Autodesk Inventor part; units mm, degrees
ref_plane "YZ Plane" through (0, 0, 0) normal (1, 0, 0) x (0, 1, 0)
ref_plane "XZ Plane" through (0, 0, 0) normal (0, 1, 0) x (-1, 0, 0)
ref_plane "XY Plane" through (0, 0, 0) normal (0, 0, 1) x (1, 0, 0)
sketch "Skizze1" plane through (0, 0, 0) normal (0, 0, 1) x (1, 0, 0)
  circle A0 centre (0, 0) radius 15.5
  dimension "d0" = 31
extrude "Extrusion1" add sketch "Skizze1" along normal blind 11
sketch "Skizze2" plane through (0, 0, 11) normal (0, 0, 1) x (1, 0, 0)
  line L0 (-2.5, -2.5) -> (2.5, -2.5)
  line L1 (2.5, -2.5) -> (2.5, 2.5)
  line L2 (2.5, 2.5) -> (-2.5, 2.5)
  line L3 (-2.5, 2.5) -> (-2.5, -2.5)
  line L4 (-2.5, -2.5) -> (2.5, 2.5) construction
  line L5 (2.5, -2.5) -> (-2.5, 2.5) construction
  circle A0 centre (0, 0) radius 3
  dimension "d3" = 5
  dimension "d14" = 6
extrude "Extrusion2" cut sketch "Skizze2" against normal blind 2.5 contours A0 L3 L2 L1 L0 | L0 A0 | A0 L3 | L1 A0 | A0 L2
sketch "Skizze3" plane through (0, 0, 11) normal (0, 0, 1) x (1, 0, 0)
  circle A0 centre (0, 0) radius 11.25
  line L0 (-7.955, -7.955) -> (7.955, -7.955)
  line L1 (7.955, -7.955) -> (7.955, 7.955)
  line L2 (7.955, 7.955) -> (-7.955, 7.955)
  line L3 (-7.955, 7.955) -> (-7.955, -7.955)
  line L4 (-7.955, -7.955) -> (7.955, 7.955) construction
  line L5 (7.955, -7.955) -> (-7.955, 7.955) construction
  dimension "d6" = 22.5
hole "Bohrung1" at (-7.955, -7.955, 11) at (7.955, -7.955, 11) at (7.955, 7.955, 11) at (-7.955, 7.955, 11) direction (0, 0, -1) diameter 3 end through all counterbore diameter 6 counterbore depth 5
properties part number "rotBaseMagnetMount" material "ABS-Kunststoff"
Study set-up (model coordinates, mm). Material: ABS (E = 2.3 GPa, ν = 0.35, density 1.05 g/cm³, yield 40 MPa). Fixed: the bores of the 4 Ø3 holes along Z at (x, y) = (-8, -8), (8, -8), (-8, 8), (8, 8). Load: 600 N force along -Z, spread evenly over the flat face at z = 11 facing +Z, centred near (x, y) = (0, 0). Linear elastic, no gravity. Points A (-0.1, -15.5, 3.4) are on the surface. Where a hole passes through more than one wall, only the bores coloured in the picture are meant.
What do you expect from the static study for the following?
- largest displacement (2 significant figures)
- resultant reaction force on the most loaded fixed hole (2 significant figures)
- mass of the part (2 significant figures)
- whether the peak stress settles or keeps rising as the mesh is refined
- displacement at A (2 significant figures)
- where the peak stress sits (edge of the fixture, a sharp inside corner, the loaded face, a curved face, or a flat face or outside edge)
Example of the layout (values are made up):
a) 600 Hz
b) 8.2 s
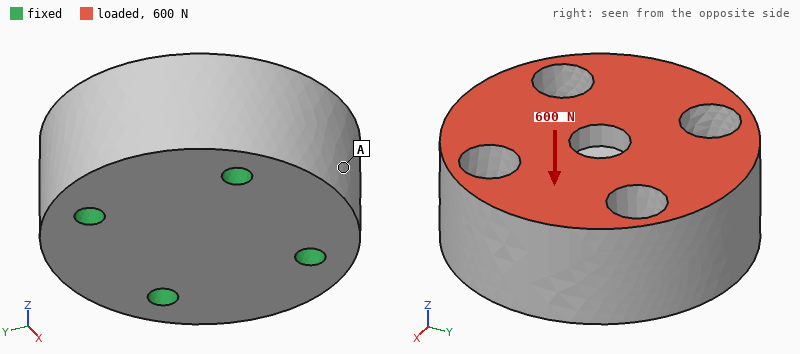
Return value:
a) 13 µm
b) 150 N
c) 7.9 g
d) keeps rising
e) 11 µm
f) edge of the fixture
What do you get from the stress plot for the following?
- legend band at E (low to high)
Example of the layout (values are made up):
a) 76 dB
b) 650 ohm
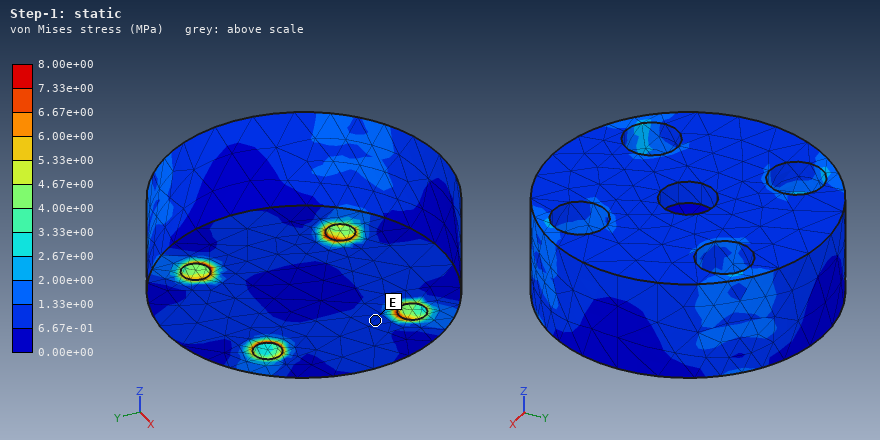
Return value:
a) 6.67e-01 to 1.33e+00 MPa
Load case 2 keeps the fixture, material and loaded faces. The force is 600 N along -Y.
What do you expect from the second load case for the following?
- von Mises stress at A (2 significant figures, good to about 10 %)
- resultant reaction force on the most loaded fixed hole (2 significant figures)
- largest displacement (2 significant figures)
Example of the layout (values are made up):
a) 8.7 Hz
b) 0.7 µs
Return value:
a) 1.0 MPa
b) 190 N
c) 37 µm
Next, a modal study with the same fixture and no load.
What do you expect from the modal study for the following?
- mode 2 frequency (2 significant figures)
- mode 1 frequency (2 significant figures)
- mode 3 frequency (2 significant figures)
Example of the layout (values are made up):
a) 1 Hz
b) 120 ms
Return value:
a) 14 kHz
b) 14 kHz
c) 15 kHz
